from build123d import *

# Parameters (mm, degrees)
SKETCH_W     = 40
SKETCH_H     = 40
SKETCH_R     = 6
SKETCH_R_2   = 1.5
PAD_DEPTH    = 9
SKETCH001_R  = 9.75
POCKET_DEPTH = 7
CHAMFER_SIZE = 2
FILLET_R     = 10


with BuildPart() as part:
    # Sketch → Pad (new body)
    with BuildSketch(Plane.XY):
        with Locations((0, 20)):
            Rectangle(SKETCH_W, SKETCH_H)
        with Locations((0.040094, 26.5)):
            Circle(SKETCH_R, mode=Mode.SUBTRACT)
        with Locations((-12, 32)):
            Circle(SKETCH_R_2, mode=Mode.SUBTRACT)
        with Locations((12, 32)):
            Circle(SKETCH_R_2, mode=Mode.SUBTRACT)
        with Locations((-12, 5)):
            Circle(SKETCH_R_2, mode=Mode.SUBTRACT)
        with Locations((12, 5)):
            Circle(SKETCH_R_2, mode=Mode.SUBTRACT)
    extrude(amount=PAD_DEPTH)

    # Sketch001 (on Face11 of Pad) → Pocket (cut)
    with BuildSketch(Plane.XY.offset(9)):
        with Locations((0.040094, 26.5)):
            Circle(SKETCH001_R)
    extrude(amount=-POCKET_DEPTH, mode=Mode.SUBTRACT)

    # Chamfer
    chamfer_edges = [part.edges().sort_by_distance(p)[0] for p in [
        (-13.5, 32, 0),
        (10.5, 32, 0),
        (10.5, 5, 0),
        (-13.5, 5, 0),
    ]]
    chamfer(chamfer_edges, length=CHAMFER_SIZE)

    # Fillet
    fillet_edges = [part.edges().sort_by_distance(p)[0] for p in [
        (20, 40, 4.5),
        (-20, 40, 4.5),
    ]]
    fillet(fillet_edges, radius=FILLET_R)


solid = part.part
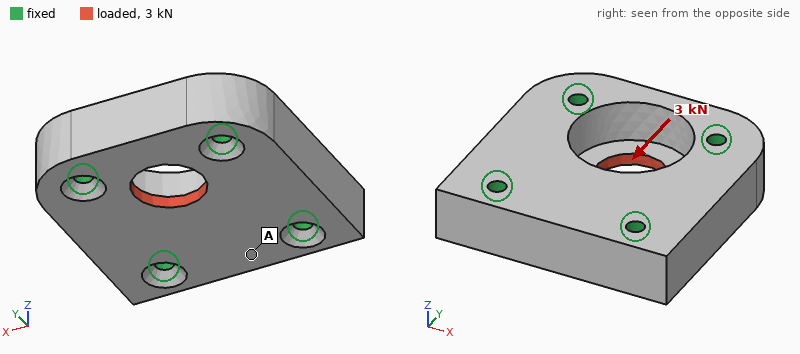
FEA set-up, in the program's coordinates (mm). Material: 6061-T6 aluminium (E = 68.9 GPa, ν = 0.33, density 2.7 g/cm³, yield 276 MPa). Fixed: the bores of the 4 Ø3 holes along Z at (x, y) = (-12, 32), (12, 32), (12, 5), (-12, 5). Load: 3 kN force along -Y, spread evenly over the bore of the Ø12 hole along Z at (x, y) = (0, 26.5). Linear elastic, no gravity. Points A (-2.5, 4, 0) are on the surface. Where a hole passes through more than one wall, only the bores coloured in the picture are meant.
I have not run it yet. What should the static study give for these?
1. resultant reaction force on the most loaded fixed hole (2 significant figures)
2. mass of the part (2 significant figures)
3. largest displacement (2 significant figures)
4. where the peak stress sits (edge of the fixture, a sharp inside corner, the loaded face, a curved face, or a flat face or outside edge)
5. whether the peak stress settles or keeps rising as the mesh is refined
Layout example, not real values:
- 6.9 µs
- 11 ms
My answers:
- 970 N
- 31 g
- 12 µm
- edge of the fixture
- keeps rising
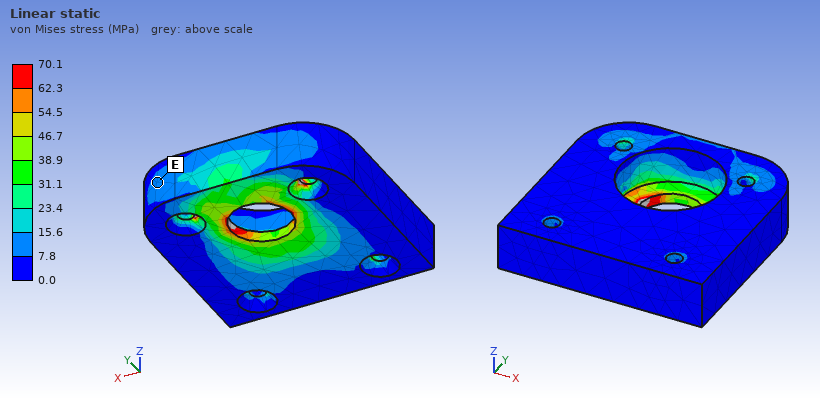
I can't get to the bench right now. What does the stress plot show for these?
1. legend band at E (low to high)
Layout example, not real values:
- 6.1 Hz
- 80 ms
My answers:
- 7.8 to 15.6 MPa
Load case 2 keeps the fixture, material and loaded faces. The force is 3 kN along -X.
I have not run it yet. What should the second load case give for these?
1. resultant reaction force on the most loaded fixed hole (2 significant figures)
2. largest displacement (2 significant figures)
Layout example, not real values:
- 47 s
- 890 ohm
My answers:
- 1.0 kN
- 8.5 µm
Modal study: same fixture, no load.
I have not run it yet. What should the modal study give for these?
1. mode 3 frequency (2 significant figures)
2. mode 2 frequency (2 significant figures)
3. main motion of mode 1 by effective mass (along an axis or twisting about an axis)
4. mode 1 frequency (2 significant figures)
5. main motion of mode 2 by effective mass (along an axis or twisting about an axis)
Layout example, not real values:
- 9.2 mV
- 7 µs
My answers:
- 36 kHz
- 34 kHz
- along Z
- 29 kHz
- twisting about Y
